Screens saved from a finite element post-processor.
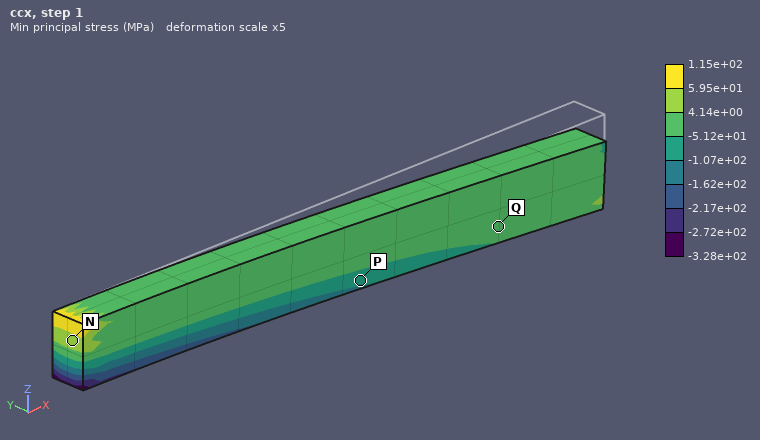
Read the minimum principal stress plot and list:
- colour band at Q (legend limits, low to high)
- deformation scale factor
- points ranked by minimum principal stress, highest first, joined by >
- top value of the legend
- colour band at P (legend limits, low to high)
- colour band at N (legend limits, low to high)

-5.12e+01 to 4.14e+00 MPa
5
N > Q > P
1.15e+02 MPa
-1.07e+02 to -5.12e+01 MPa
4.14e+00 to 5.95e+01 MPa
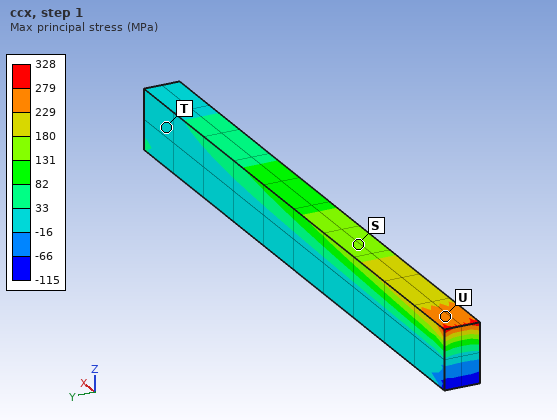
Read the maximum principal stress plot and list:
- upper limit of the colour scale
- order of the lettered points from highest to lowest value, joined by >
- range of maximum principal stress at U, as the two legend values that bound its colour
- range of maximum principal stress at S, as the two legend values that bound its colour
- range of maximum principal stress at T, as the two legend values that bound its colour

328 MPa
U > S > T
229 to 279 MPa
131 to 180 MPa
-16 to 33 MPa
